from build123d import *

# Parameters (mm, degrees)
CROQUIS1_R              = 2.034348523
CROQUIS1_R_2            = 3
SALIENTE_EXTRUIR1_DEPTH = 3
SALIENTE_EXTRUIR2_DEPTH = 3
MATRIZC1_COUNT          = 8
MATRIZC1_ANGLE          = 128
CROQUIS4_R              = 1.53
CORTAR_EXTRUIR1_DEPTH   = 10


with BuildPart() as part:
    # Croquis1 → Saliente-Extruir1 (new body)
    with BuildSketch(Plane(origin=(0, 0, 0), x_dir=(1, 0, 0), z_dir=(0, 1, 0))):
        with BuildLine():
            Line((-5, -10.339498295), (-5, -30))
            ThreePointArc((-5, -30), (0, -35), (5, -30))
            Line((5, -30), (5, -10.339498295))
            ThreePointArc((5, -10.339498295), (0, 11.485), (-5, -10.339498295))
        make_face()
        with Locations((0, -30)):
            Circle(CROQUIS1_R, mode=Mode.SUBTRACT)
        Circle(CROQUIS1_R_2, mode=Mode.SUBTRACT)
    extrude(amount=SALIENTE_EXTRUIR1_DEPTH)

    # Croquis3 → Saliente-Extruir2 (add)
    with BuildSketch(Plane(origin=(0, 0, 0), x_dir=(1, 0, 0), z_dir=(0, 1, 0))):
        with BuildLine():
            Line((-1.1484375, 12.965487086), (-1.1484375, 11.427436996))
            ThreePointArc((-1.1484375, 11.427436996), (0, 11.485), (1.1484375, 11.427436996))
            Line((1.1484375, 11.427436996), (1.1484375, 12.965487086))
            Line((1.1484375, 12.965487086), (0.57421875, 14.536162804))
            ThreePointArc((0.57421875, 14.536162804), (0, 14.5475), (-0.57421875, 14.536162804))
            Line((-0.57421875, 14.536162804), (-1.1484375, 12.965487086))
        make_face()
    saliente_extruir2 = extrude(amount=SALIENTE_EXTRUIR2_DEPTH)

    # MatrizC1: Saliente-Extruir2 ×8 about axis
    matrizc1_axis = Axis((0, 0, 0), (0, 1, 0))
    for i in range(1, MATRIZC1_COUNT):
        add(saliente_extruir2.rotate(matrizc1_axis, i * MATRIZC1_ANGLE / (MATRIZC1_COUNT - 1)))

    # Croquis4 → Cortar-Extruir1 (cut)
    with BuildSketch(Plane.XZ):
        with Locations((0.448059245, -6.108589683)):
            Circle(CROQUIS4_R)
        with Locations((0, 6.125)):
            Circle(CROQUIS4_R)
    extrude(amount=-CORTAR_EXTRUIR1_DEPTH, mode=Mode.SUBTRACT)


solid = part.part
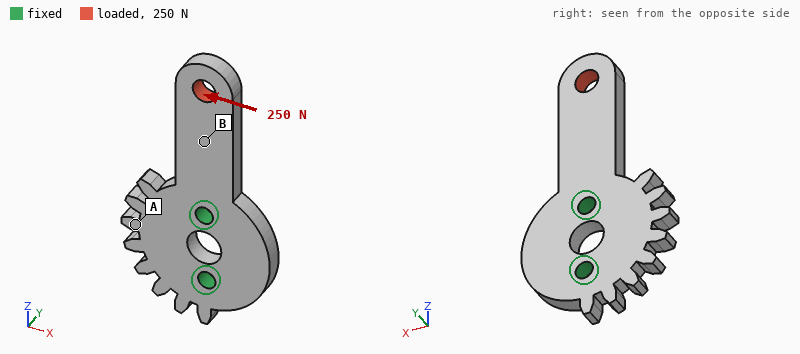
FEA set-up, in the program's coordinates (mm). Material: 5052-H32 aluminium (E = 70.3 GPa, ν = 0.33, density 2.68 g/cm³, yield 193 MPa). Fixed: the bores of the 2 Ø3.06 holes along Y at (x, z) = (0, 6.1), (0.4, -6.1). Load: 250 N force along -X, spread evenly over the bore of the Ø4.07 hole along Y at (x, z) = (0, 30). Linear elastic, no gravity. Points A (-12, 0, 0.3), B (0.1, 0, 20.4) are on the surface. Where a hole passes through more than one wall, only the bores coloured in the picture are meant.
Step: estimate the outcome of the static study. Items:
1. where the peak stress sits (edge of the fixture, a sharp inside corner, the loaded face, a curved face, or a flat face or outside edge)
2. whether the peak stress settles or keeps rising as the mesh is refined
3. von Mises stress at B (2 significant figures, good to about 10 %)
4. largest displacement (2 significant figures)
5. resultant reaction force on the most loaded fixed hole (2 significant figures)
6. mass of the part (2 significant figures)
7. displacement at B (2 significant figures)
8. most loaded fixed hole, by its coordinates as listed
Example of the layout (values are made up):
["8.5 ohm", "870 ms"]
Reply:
["a sharp inside corner", "keeps rising", "22 MPa", "97 µm", "530 N", "5.1 g", "33 µm", "(0, 6.1)"]
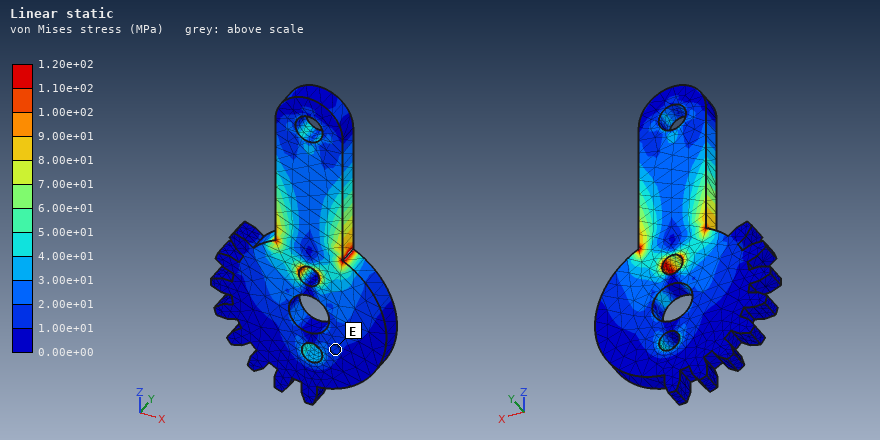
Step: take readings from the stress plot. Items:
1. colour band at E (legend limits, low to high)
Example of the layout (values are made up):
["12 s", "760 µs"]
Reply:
["1.00e+01 to 2.00e+01 MPa"]
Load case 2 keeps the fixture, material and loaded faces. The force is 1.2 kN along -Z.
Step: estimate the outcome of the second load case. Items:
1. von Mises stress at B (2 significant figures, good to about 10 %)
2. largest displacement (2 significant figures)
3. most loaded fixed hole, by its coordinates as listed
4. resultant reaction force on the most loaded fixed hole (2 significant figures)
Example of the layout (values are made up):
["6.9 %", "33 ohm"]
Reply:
["39 MPa", "18 µm", "(0, 6.1)", "1.0 kN"]
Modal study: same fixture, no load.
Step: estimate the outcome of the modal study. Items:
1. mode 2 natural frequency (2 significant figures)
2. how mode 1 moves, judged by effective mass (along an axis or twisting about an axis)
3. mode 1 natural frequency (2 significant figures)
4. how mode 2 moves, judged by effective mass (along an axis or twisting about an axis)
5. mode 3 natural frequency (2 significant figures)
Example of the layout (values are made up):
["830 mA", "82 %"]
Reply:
["10 kHz", "along Y", "3700 Hz", "along X", "16 kHz"]
